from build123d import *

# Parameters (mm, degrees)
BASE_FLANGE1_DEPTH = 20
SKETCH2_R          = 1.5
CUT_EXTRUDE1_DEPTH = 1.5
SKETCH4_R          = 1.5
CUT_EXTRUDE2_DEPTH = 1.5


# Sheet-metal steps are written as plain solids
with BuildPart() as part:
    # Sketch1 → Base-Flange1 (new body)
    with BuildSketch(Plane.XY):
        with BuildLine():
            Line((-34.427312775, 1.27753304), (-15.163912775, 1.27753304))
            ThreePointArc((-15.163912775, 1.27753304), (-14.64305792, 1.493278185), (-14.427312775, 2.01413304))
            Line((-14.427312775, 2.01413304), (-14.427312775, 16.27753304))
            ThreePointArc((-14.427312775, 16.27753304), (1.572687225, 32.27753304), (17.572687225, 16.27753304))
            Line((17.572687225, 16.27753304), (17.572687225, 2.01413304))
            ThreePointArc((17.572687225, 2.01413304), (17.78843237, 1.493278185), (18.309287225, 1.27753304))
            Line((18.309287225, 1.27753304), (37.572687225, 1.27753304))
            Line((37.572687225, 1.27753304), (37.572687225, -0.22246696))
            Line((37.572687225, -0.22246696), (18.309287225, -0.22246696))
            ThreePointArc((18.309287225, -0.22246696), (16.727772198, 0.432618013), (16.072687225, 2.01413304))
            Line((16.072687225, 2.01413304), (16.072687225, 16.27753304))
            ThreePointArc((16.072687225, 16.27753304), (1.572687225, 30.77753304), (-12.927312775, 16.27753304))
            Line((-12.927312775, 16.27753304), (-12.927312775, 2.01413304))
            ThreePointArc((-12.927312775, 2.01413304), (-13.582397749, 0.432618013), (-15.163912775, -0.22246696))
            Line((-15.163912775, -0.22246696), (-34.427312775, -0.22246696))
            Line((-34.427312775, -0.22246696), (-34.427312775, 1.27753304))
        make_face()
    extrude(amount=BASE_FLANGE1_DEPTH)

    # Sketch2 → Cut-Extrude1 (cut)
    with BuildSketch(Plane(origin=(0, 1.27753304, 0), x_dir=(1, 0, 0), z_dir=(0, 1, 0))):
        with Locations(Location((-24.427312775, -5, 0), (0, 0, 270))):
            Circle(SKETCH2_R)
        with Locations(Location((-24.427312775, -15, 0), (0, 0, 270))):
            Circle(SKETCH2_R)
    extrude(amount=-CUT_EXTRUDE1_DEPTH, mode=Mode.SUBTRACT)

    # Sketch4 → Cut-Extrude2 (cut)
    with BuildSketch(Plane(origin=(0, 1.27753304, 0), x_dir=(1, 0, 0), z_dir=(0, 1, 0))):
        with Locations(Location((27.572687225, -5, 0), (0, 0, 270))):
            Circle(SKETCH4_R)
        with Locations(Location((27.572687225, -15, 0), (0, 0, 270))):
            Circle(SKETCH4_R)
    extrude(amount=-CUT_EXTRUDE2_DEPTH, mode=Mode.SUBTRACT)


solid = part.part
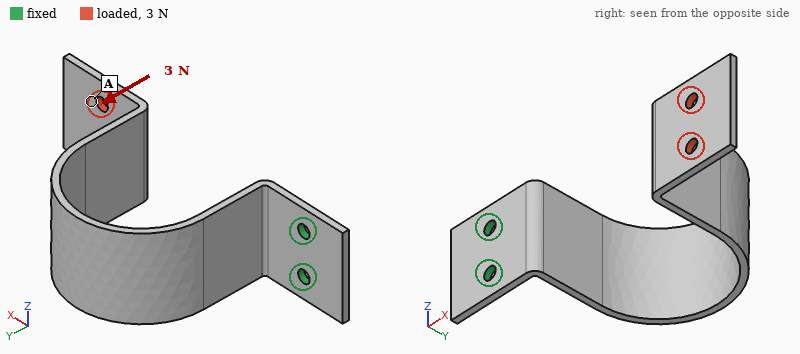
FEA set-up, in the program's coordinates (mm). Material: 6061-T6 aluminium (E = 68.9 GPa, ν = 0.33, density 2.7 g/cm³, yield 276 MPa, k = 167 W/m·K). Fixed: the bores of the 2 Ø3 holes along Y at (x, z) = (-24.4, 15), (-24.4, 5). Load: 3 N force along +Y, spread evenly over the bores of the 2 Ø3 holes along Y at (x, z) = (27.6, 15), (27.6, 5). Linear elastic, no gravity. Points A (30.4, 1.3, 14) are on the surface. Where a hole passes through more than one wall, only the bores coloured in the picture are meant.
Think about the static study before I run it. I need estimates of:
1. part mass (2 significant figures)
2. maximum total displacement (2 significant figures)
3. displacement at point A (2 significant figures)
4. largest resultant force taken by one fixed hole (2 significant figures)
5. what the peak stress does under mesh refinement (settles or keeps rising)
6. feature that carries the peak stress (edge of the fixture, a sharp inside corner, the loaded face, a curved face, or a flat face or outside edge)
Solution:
9.6 g
0.87 mm
0.73 mm
2.2 N
keeps rising
edge of the fixture
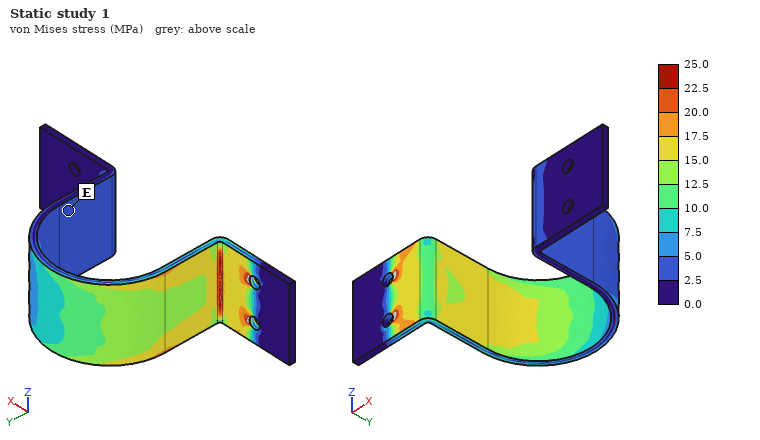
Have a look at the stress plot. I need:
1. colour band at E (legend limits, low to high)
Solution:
2.5 to 5.0 MPa
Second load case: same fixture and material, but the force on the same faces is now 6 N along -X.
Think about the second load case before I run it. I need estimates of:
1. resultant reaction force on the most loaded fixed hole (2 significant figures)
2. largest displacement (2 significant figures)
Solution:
3.0 N
0.92 mm
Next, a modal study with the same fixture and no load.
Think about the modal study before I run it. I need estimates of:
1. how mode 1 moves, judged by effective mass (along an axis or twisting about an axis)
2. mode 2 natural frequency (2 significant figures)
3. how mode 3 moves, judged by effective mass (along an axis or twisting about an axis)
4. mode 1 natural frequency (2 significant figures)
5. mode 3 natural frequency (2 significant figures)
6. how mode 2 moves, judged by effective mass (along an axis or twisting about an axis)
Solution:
along Y
270 Hz
along X
180 Hz
390 Hz
along Z
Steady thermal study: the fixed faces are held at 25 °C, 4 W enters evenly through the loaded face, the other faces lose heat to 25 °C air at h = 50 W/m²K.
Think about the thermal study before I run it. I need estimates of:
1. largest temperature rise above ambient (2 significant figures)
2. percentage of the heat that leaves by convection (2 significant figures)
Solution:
32 K
79 %
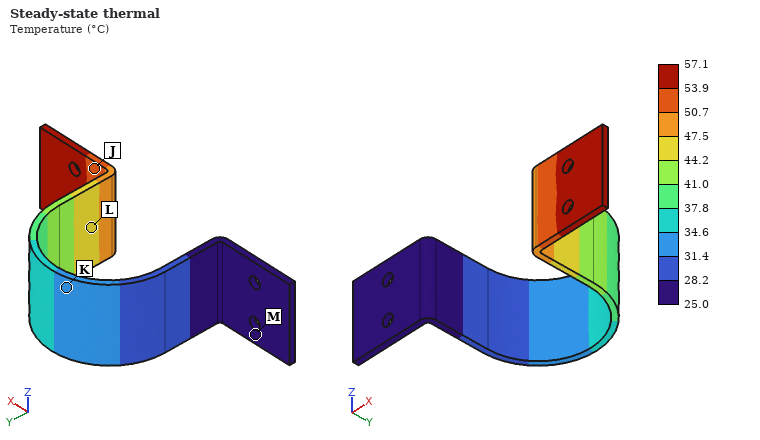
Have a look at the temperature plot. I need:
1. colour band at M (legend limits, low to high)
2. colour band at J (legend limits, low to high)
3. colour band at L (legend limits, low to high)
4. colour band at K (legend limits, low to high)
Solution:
25.0 to 28.2 °C
50.7 to 53.9 °C
44.2 to 47.5 °C
31.4 to 34.6 °C
